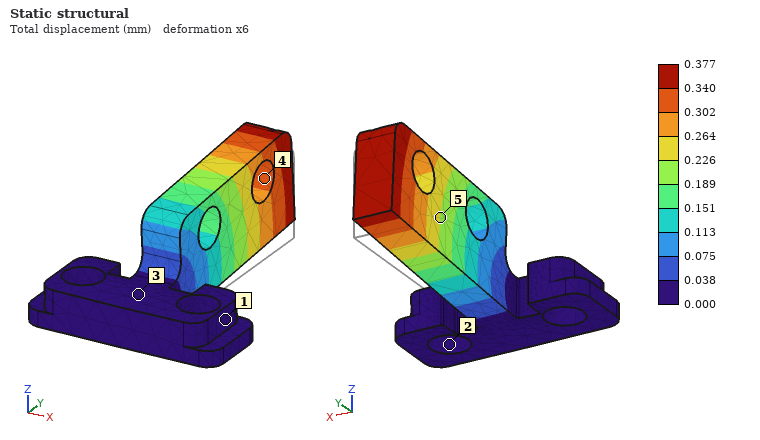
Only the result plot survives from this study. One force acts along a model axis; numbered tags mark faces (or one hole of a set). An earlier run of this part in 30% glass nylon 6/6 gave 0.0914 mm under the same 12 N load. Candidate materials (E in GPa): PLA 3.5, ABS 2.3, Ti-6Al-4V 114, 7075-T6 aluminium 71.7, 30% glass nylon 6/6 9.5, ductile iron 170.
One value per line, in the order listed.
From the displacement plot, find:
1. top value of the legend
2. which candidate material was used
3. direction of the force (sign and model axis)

0.377 mm
ABS
+Z
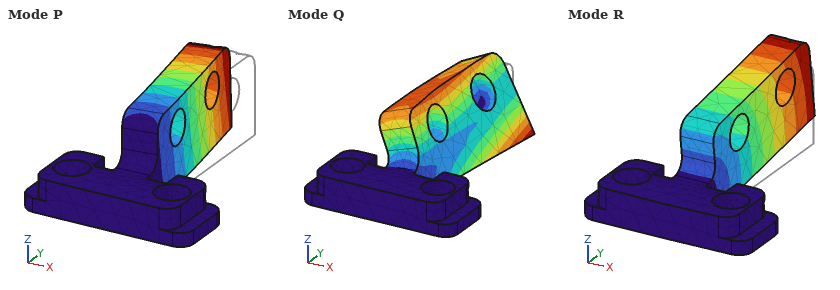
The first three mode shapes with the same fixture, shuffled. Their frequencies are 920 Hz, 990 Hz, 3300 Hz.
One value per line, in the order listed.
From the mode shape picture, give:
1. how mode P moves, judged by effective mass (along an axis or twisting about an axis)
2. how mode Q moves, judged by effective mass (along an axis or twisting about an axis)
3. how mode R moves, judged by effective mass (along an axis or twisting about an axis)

along X
twisting about Y
along Z
